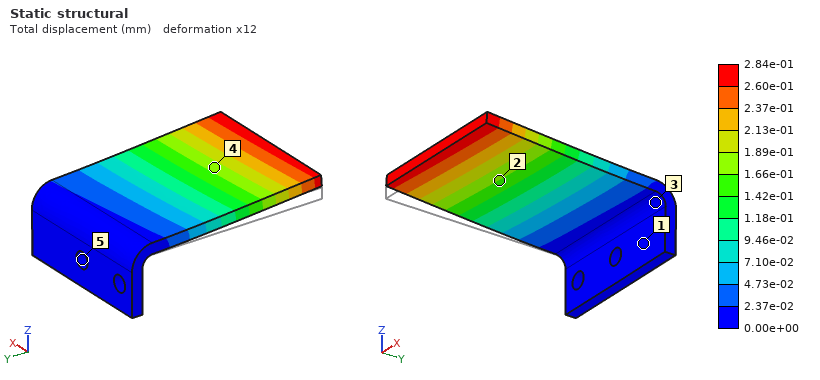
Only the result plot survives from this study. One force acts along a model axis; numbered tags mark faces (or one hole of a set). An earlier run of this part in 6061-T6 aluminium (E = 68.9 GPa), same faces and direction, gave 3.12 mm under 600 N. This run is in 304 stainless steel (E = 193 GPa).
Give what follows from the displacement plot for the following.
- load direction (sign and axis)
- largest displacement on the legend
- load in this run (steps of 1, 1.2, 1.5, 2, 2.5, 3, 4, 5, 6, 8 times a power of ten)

+Z
2.84e-01 mm
150 N
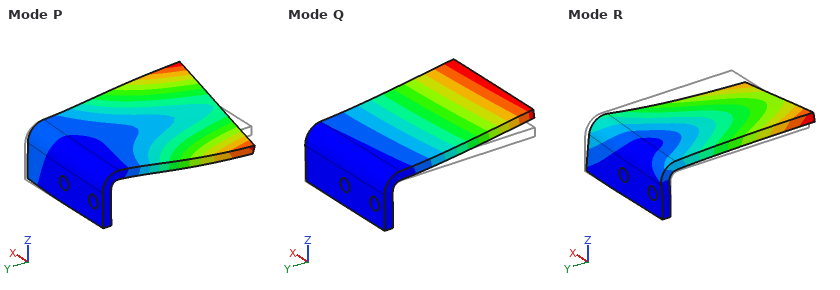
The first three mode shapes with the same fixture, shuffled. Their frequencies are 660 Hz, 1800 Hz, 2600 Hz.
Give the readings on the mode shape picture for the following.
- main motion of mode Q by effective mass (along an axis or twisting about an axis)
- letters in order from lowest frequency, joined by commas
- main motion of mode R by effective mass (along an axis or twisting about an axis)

along Z
Q, R, P
along X
